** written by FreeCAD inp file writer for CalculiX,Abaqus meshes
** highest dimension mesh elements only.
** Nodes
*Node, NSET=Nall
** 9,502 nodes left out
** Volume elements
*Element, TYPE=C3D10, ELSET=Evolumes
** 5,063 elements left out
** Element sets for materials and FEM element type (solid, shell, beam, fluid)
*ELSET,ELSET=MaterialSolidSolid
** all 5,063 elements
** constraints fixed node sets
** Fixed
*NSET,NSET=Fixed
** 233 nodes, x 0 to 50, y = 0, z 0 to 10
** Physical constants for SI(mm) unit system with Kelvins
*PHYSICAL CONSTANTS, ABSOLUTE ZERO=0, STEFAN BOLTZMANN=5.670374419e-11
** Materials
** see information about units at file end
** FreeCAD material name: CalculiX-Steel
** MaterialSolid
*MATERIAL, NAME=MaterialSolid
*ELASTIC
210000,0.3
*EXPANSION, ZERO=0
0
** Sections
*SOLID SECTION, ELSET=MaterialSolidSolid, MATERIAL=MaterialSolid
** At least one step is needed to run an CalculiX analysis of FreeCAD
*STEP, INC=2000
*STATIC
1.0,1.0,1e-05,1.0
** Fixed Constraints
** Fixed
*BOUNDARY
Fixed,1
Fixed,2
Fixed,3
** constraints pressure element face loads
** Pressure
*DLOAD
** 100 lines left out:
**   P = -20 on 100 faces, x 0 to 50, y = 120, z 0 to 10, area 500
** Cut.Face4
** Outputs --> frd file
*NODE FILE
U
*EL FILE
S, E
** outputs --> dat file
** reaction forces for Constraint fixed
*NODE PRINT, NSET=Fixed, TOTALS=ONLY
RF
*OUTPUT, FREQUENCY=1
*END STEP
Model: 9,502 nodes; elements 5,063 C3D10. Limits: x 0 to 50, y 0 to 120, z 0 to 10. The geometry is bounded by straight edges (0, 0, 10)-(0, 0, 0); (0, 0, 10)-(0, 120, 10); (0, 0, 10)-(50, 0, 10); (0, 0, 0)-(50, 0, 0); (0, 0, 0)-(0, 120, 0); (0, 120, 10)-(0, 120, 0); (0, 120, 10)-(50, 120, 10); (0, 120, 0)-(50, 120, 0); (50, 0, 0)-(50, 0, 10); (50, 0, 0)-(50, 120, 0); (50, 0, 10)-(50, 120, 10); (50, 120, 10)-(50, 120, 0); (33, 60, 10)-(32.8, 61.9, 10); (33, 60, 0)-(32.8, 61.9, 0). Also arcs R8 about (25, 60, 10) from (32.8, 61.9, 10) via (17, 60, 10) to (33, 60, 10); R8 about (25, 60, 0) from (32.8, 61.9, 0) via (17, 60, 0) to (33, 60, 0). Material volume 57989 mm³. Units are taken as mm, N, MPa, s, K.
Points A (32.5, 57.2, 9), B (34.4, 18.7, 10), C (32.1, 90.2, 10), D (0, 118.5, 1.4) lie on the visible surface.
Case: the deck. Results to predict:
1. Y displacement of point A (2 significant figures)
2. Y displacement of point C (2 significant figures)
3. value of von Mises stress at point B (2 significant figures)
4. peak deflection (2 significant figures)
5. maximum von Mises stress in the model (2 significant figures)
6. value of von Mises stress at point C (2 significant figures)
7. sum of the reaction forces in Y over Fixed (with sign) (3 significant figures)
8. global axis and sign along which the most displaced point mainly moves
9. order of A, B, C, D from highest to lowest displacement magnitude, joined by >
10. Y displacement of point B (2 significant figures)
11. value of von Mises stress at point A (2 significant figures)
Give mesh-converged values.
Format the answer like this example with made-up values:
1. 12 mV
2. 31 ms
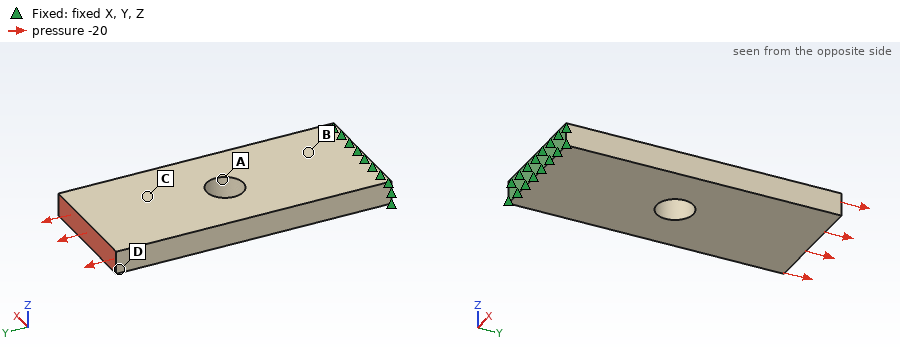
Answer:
1. 0.0054 mm
2. 0.0099 mm
3. 19 MPa
4. 0.013 mm
5. 70 MPa
6. 18 MPa
7. -10000 N
8. +Y
9. D > C > A > B
10. 0.0016 mm
11. 56 MPa
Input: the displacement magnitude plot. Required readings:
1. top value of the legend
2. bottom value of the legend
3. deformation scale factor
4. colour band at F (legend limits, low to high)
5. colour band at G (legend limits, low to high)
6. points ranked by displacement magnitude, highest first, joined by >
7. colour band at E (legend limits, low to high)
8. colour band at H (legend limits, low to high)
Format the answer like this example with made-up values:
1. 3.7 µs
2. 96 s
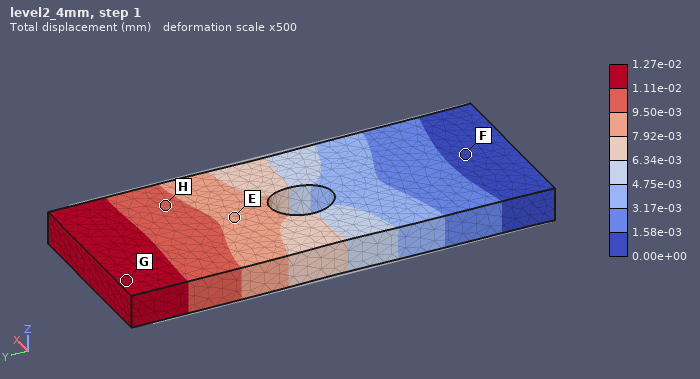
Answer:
1. 1.27e-02 mm
2. 0.00e+00 mm
3. 500
4. 0.00e+00 to 1.58e-03 mm
5. 1.11e-02 to 1.27e-02 mm
6. G > H > E > F
7. 7.92e-03 to 9.50e-03 mm
8. 9.50e-03 to 1.11e-02 mm
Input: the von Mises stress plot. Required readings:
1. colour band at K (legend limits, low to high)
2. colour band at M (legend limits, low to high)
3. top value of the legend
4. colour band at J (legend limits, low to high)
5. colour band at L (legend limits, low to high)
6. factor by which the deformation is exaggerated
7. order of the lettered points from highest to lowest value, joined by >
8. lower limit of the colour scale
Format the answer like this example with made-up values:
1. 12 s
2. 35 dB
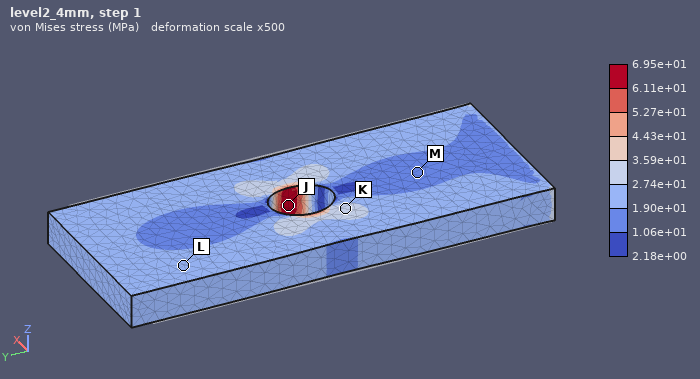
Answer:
1. 2.74e+01 to 3.59e+01 MPa
2. 1.06e+01 to 1.90e+01 MPa
3. 6.95e+01 MPa
4. 6.11e+01 to 6.95e+01 MPa
5. 1.90e+01 to 2.74e+01 MPa
6. 500
7. J > K > L > M
8. 2.18e+00 MPa
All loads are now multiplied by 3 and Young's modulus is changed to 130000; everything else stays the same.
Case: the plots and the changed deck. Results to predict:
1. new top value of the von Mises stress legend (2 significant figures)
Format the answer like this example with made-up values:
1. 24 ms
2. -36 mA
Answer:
1. 210 MPa
